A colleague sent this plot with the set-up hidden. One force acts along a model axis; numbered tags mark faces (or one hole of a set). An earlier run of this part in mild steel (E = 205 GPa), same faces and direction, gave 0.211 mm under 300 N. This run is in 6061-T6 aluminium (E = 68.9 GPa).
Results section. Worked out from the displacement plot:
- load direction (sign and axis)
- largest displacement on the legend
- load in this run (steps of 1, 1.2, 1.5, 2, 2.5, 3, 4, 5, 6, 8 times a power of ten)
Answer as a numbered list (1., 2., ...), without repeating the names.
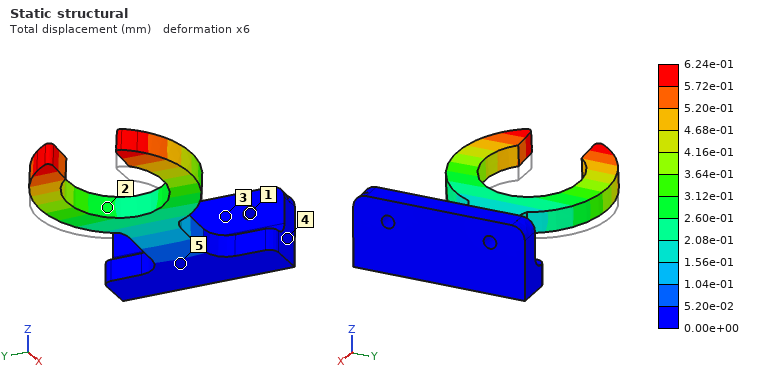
1. +Z
2. 6.24e-01 mm
3. 300 N
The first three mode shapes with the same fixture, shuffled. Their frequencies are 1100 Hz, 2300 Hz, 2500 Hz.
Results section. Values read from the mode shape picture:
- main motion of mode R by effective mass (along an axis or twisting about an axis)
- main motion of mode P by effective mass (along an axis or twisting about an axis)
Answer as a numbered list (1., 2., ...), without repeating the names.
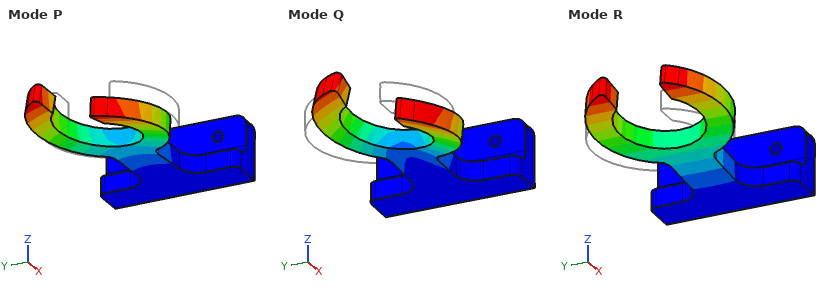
1. along Z
2. along Y
